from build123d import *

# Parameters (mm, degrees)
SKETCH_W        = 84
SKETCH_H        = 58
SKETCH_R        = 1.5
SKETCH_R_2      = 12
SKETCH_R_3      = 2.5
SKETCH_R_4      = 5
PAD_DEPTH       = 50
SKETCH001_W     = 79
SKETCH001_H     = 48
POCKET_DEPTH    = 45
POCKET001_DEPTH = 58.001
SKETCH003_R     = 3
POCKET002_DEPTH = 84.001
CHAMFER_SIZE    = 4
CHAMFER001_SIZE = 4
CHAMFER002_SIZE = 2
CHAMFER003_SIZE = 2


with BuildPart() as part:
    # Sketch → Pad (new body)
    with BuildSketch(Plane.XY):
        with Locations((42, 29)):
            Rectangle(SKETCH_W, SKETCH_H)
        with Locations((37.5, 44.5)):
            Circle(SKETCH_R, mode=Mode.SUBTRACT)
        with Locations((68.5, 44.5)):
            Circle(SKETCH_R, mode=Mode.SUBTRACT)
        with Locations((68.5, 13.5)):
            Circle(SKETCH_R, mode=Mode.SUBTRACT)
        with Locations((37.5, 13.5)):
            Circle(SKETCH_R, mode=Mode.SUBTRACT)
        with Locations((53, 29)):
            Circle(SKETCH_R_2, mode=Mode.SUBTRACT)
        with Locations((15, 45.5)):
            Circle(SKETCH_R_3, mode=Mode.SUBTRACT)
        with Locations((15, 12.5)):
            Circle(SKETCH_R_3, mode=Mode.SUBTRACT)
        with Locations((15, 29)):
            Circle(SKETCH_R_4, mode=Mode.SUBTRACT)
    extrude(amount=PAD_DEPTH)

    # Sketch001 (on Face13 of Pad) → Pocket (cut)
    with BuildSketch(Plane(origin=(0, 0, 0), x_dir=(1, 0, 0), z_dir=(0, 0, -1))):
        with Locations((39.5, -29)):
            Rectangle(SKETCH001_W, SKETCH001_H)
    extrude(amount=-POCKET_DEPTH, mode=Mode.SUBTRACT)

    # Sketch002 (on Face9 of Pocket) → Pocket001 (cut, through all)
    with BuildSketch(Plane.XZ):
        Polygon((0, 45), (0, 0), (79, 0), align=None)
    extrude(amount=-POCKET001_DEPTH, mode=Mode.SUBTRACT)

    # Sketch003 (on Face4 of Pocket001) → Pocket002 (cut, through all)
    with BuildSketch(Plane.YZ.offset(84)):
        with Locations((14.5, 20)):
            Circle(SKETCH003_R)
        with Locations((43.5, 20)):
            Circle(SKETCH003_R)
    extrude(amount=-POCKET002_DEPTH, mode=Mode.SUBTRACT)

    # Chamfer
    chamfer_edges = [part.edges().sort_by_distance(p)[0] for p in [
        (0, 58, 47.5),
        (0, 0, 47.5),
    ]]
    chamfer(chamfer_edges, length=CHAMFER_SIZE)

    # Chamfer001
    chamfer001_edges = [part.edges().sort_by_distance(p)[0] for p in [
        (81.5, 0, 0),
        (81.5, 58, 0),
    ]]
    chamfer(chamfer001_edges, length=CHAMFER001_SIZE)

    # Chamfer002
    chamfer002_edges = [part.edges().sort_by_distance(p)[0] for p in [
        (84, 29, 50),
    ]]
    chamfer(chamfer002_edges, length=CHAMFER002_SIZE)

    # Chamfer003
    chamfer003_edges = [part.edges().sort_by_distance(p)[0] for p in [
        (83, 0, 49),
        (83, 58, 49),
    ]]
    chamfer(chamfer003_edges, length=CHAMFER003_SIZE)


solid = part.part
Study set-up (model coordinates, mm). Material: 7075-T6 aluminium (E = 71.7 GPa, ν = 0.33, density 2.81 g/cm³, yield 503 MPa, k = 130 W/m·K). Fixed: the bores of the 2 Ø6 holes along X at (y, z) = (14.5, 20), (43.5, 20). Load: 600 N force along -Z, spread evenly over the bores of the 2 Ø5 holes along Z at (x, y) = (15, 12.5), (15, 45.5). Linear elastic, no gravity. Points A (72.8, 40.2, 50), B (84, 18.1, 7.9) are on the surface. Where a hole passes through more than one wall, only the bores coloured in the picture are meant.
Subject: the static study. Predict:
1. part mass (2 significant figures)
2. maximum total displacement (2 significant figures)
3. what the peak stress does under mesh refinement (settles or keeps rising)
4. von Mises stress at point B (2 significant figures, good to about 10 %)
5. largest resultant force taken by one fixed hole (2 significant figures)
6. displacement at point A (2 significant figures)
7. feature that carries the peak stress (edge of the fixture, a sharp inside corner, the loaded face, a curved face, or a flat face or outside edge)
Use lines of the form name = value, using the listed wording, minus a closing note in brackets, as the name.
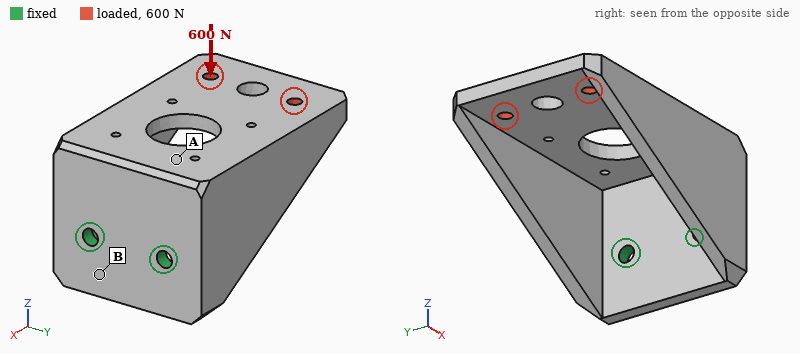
part mass = 140 g
maximum total displacement = 0.40 mm
what the peak stress does under mesh refinement = keeps rising
von Mises stress at point B = 40 MPa
largest resultant force taken by one fixed hole = 320 N
displacement at point A = 0.12 mm
feature that carries the peak stress = edge of the fixture
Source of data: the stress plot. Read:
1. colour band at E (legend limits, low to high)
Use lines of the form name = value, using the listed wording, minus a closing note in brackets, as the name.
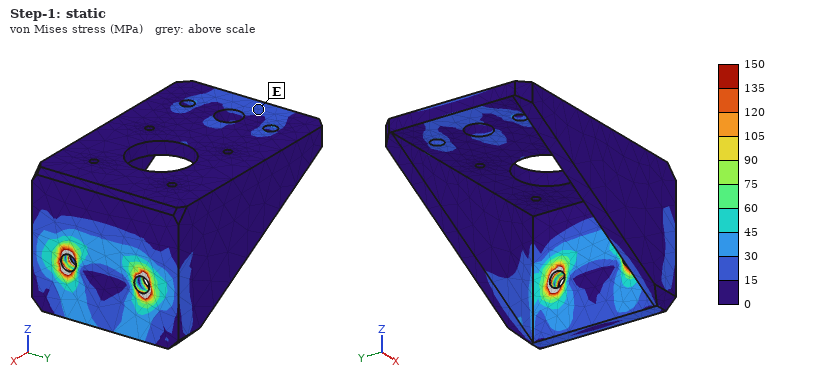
colour band at E = 15 to 30 MPa
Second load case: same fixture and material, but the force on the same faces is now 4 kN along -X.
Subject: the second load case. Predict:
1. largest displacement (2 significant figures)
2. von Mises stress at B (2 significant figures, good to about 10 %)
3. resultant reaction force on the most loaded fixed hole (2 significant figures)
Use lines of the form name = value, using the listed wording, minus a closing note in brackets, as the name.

largest displacement = 0.94 mm
von Mises stress at B = 77 MPa
resultant reaction force on the most loaded fixed hole = 2.0 kN
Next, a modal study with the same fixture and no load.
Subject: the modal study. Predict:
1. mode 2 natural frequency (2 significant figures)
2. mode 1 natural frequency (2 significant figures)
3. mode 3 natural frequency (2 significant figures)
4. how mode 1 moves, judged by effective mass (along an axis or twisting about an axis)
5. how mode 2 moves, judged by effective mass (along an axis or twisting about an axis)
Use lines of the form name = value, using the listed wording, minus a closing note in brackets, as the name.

mode 2 natural frequency = 1100 Hz
mode 1 natural frequency = 990 Hz
mode 3 natural frequency = 3800 Hz
how mode 1 moves, judged by effective mass = along Z
how mode 2 moves, judged by effective mass = along Y
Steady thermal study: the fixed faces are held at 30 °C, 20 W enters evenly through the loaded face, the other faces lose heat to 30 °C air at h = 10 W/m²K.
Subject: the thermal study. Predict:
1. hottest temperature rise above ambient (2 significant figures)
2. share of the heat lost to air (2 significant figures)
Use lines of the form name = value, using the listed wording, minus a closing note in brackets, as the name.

hottest temperature rise above ambient = 30 K
share of the heat lost to air = 14 %
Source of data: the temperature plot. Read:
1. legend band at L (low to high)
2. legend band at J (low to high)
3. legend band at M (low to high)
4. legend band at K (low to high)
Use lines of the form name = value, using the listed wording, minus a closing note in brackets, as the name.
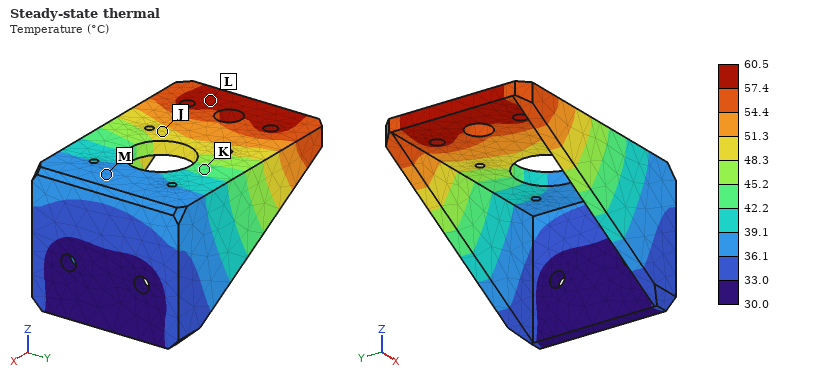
legend band at L = 57.4 to 60.5 °C
legend band at J = 48.3 to 51.3 °C
legend band at M = 36.1 to 39.1 °C
legend band at K = 42.2 to 45.2 °C
